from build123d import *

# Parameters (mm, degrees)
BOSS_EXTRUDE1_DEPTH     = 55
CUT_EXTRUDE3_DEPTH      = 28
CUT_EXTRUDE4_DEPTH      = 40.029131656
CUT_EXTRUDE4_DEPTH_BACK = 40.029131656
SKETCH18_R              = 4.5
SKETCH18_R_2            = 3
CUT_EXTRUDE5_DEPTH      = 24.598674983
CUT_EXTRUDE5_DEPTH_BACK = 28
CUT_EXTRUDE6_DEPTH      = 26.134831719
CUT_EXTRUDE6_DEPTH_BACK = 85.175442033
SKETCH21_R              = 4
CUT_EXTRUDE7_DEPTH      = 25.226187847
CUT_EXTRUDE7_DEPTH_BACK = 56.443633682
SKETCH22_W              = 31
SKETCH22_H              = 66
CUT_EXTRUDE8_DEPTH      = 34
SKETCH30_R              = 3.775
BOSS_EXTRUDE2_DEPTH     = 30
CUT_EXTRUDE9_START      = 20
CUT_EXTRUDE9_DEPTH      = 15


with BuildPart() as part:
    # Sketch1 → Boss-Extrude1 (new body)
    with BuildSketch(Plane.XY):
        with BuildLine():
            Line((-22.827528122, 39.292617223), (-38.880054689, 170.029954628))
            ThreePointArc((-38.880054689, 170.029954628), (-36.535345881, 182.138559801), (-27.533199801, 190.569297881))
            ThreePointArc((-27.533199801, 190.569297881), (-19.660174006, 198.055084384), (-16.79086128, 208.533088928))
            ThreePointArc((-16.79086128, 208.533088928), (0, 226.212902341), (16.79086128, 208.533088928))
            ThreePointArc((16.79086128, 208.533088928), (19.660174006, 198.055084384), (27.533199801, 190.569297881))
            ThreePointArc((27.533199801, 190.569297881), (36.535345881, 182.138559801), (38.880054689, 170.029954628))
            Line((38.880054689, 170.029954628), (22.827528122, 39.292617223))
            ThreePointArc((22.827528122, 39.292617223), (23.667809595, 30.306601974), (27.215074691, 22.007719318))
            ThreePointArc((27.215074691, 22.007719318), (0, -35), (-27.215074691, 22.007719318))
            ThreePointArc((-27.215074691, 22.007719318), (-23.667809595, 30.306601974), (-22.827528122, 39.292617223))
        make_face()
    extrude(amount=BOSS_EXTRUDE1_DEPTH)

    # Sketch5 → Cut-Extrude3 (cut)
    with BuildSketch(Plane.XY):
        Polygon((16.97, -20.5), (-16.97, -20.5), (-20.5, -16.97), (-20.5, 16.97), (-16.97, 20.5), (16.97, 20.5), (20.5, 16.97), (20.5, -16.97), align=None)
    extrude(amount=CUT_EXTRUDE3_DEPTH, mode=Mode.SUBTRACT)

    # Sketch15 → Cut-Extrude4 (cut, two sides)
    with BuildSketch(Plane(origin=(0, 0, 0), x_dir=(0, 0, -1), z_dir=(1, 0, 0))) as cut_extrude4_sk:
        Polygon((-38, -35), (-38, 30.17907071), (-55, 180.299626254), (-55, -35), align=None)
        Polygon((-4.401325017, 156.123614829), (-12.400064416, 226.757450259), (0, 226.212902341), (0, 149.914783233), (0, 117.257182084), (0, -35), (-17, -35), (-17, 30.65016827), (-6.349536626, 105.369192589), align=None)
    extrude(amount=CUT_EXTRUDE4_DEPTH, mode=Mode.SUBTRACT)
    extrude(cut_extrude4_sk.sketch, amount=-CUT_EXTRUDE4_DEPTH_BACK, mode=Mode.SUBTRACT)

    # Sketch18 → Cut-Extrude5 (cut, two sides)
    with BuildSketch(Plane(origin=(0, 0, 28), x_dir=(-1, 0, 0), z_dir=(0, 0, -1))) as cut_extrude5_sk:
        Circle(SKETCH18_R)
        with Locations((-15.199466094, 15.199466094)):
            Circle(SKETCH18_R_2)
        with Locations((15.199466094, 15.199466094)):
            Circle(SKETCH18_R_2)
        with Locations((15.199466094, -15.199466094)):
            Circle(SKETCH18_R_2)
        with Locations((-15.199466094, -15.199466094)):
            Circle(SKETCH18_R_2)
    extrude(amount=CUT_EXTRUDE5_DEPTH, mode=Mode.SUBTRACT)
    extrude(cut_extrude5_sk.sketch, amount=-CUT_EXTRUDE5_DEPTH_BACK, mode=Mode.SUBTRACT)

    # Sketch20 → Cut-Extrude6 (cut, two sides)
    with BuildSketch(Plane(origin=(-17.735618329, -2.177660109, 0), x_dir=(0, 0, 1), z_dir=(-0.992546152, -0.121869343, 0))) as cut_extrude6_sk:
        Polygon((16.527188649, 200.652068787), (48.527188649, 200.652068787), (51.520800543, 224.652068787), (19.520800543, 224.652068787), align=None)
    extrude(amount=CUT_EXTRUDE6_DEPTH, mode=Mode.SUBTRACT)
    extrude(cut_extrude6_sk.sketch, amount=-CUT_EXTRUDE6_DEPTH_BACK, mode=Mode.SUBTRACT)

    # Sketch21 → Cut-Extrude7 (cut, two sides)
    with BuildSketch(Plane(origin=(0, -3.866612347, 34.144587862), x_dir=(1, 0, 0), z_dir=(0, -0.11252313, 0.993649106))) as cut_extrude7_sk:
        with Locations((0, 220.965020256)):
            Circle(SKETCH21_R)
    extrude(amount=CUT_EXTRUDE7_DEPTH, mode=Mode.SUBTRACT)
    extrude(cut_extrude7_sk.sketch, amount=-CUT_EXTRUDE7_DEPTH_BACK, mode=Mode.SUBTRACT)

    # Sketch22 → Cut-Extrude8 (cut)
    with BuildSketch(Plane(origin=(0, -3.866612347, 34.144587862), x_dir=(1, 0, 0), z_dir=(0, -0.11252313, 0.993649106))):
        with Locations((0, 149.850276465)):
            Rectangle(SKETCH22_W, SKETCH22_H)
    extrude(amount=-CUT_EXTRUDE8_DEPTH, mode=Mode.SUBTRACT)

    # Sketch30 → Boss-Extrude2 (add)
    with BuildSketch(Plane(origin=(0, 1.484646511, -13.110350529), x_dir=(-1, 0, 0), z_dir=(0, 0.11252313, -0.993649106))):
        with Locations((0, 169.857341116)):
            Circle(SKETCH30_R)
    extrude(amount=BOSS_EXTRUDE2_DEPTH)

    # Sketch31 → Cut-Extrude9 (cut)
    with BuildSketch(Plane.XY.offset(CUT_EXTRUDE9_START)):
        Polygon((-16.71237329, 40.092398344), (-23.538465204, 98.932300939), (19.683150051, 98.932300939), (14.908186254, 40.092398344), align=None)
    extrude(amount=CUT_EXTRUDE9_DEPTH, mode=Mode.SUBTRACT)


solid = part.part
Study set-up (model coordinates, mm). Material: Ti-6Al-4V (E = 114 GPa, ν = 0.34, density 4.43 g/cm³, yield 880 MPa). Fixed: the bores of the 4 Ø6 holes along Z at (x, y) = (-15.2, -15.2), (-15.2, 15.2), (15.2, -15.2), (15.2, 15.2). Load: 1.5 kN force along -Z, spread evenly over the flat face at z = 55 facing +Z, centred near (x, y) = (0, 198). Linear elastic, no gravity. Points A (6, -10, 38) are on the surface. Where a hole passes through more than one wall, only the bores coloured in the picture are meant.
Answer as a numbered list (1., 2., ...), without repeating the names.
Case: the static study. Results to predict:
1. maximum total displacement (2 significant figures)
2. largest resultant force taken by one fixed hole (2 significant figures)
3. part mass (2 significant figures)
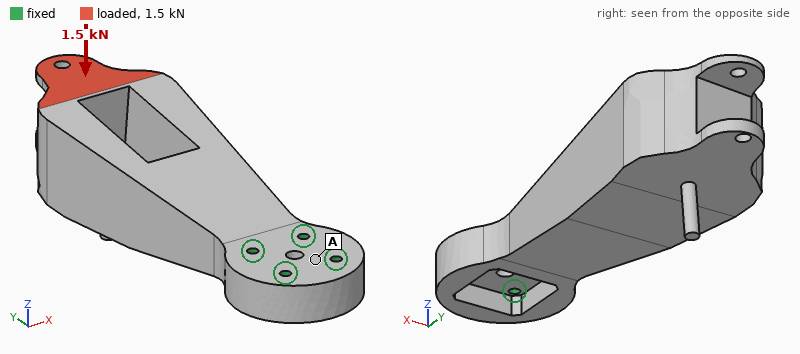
1. 0.90 mm
2. 4.1 kN
3. 1.7 kg
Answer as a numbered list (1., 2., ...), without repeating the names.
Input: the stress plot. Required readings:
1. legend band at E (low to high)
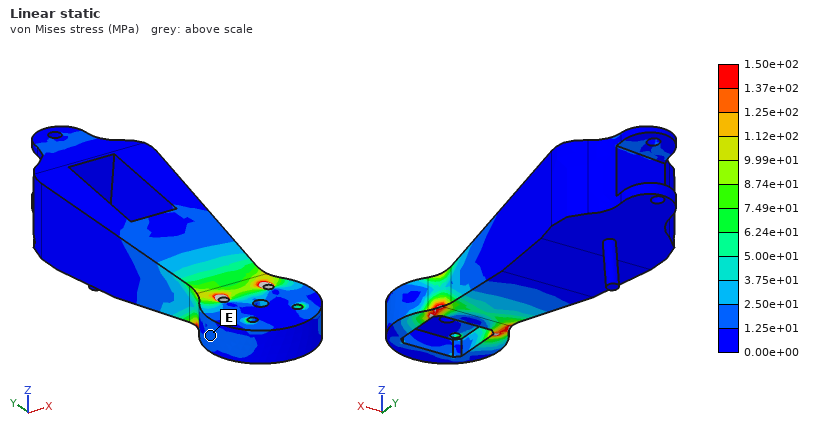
1. 1.25e+01 to 2.50e+01 MPa
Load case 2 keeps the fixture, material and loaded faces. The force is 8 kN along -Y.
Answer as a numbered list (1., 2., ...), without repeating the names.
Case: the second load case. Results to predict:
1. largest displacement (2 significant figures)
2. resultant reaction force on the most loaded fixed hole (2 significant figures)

1. 0.79 mm
2. 4.9 kN
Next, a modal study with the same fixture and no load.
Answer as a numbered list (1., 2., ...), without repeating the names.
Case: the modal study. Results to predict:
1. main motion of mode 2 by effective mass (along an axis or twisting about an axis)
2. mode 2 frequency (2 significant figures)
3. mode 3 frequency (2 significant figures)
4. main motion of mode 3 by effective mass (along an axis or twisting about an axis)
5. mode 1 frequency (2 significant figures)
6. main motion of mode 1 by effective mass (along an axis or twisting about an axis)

1. along X
2. 640 Hz
3. 1500 Hz
4. twisting about Y
5. 270 Hz
6. along Z
